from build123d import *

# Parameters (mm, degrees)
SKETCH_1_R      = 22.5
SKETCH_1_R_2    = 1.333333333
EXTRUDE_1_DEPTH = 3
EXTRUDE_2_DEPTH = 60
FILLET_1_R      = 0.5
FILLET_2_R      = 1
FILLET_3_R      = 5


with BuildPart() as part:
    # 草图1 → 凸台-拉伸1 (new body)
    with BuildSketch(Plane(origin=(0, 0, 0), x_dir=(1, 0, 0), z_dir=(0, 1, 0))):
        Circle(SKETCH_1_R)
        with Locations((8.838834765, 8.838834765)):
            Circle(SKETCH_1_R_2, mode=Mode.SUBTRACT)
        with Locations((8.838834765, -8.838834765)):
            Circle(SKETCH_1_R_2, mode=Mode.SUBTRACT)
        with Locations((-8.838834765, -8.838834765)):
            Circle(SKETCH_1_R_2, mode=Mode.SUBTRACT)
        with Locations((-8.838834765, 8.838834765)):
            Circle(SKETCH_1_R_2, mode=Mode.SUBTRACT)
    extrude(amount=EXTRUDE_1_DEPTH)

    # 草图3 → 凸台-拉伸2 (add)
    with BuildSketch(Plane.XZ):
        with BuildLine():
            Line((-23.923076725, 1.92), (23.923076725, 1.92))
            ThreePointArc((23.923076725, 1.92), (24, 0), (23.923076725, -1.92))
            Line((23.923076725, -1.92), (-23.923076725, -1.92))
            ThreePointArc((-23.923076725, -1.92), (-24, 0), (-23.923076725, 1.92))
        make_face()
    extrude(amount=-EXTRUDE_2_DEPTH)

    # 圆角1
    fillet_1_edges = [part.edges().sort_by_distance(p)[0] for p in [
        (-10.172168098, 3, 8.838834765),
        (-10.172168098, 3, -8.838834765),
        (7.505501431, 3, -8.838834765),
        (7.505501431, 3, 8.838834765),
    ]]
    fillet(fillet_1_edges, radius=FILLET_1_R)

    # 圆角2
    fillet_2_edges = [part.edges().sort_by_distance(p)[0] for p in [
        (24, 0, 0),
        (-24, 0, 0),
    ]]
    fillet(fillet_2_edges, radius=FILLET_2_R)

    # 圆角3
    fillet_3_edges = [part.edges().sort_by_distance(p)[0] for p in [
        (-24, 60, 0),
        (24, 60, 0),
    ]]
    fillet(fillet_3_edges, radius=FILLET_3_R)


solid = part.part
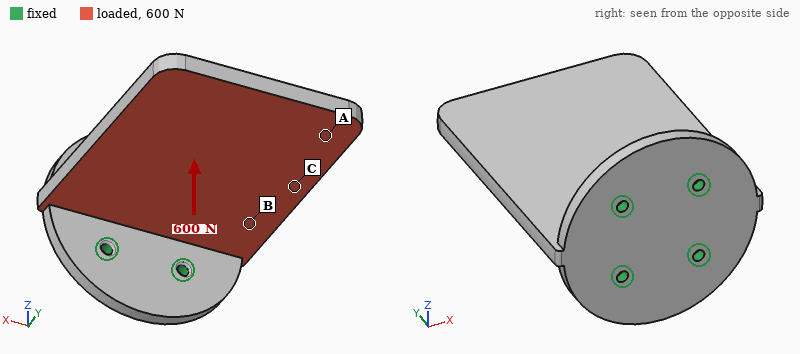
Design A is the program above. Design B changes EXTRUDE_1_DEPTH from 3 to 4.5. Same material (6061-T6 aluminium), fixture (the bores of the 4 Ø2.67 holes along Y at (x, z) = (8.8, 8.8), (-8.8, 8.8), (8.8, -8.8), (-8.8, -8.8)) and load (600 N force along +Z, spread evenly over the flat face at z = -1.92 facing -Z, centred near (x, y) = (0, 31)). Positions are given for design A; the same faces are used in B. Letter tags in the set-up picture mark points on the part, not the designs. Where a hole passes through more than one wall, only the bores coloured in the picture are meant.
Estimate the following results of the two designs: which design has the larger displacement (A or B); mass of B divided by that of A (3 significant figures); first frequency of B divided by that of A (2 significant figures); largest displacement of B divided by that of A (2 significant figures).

A
1.14
1.1
0.84
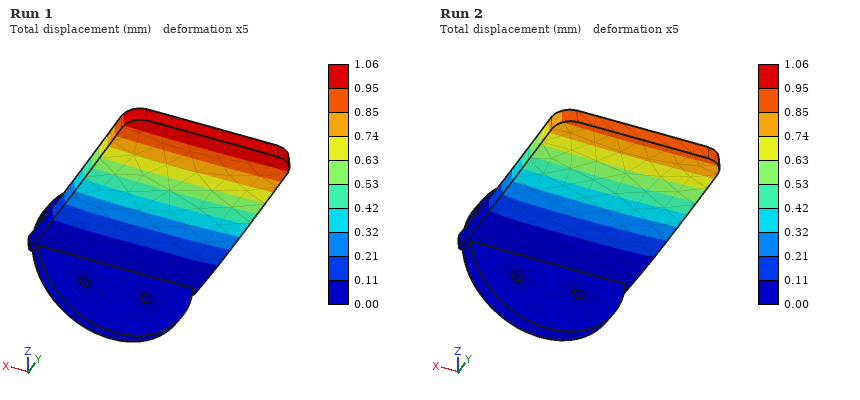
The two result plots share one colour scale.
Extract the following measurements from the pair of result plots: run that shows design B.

Run 2
